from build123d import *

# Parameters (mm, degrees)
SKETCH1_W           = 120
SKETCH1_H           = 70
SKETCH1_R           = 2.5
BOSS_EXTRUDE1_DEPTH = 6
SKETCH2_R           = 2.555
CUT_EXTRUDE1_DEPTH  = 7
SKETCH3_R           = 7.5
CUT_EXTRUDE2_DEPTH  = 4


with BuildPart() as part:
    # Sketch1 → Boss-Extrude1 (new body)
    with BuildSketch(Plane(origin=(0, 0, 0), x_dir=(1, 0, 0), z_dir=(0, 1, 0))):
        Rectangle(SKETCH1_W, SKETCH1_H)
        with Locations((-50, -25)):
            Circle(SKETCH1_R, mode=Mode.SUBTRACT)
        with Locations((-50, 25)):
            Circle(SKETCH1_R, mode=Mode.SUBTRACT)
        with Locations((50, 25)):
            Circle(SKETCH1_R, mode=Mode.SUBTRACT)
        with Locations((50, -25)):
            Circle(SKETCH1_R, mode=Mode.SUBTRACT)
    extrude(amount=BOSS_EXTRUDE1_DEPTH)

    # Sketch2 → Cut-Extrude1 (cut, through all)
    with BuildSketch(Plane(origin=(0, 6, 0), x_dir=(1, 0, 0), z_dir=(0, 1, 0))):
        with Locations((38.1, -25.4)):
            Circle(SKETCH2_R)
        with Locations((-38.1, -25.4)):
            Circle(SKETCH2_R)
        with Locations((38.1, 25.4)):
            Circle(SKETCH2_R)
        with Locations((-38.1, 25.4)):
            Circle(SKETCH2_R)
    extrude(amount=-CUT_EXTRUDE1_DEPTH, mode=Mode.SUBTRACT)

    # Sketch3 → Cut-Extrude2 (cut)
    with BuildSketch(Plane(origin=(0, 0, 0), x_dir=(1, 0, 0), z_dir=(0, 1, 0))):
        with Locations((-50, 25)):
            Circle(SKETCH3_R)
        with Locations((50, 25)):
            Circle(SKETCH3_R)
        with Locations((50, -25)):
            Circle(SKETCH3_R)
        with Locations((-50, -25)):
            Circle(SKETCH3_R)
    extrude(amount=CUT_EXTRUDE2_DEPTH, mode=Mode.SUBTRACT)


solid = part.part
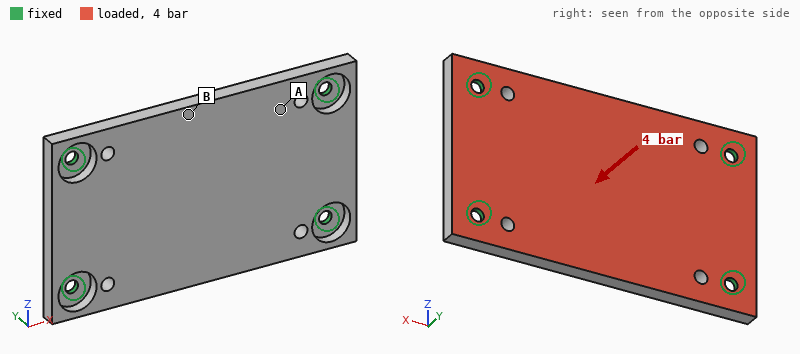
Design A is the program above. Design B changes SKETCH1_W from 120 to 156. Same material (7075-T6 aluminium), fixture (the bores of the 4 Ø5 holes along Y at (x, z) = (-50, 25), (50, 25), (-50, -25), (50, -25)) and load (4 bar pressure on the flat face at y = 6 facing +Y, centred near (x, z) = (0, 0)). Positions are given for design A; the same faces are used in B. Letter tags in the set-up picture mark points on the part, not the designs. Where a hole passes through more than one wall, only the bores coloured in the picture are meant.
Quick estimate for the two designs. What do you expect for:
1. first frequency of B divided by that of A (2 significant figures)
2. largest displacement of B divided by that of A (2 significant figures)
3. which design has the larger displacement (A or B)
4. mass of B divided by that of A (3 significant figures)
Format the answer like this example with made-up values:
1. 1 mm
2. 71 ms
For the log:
1. 0.95
2. 0.80
3. A
4. 1.32
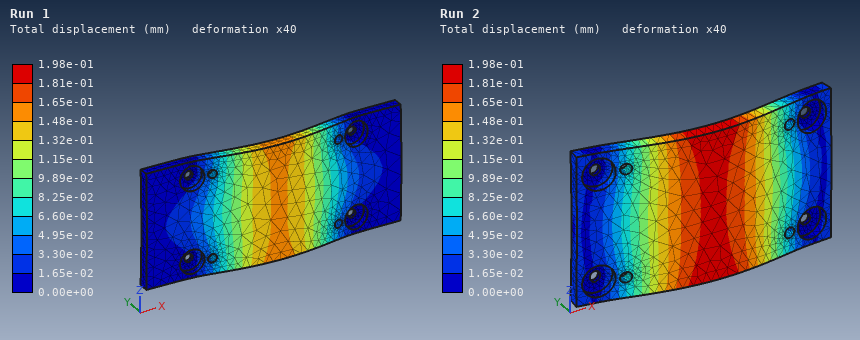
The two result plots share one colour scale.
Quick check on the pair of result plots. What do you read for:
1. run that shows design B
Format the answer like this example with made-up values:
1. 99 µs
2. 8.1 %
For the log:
1. Run 1
